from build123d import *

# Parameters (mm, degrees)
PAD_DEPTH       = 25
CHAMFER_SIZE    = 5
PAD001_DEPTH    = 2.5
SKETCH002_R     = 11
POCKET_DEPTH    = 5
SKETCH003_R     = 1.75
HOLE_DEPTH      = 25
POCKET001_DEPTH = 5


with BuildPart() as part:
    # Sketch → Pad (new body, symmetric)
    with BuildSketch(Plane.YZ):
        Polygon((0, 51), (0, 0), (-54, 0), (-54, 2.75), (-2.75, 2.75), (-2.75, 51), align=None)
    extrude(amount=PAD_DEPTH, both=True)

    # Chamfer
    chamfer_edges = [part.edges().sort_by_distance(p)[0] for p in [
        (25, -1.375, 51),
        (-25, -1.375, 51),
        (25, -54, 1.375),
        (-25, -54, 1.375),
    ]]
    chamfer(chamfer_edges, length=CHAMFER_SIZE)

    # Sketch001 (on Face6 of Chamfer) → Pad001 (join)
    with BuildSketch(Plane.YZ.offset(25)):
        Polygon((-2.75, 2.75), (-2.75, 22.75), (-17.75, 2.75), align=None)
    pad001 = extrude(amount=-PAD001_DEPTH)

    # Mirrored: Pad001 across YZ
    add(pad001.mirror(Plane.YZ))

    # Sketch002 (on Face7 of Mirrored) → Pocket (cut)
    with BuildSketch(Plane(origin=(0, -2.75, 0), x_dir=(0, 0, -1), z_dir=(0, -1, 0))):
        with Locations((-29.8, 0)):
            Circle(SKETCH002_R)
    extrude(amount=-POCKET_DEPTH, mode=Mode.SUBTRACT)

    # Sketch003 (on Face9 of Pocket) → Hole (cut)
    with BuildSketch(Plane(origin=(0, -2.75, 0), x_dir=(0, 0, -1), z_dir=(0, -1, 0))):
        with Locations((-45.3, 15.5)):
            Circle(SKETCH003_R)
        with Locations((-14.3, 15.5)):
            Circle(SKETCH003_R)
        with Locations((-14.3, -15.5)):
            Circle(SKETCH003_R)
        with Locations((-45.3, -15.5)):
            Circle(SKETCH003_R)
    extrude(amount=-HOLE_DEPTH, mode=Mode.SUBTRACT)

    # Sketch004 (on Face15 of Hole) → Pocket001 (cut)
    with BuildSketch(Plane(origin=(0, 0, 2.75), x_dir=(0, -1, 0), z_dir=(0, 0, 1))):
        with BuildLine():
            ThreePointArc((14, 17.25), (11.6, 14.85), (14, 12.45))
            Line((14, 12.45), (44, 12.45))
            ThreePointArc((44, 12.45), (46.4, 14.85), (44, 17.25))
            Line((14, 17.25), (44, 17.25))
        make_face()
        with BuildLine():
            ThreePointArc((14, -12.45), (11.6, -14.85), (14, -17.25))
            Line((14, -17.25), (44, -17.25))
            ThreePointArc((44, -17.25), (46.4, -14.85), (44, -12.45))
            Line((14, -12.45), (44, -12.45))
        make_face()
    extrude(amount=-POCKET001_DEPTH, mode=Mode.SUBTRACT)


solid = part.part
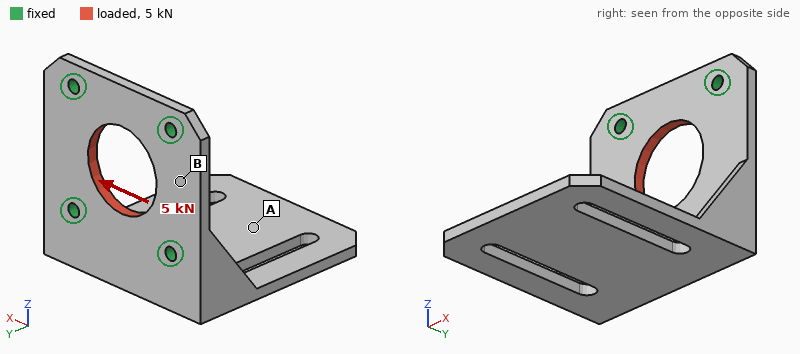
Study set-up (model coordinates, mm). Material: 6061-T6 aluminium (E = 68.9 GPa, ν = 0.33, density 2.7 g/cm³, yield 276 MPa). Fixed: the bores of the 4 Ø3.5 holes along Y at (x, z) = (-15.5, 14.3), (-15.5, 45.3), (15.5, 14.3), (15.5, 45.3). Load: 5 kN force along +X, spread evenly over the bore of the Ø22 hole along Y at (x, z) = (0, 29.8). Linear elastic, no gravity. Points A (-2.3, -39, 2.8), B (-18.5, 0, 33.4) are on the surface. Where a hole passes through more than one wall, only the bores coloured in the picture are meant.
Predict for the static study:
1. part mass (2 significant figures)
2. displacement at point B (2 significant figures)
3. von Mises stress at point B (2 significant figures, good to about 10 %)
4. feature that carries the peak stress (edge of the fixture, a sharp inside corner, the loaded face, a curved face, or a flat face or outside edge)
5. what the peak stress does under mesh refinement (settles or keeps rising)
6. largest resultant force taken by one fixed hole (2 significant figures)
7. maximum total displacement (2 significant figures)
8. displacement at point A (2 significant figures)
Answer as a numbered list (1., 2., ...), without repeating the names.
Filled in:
1. 34 g
2. 9.8 µm
3. 18 MPa
4. edge of the fixture
5. keeps rising
6. 1.3 kN
7. 12 µm
8. 2.2 µm
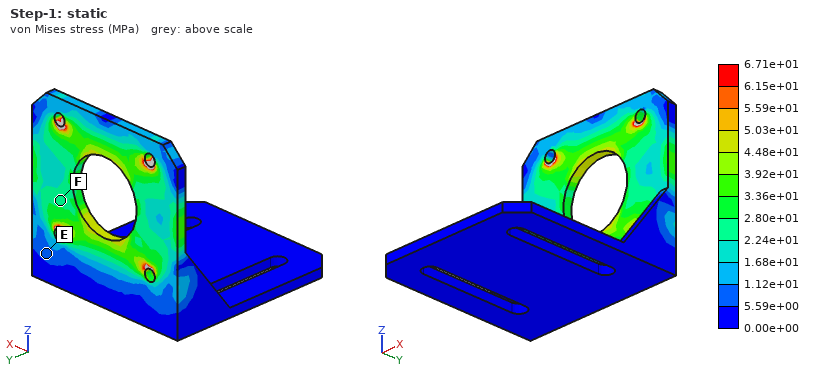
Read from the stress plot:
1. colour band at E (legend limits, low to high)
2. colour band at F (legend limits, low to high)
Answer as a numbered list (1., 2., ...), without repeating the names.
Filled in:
1. 5.59e+00 to 1.12e+01 MPa
2. 2.24e+01 to 2.80e+01 MPa
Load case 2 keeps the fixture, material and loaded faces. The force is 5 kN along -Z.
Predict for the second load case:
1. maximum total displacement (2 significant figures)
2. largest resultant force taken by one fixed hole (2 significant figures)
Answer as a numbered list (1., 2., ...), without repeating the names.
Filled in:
1. 16 µm
2. 1.3 kN
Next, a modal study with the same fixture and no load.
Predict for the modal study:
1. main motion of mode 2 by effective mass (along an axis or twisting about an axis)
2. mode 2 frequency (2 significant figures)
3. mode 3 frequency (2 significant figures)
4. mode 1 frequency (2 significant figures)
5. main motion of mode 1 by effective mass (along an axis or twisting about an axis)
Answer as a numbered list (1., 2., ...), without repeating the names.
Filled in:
1. along X
2. 2000 Hz
3. 3000 Hz
4. 880 Hz
5. along Z
